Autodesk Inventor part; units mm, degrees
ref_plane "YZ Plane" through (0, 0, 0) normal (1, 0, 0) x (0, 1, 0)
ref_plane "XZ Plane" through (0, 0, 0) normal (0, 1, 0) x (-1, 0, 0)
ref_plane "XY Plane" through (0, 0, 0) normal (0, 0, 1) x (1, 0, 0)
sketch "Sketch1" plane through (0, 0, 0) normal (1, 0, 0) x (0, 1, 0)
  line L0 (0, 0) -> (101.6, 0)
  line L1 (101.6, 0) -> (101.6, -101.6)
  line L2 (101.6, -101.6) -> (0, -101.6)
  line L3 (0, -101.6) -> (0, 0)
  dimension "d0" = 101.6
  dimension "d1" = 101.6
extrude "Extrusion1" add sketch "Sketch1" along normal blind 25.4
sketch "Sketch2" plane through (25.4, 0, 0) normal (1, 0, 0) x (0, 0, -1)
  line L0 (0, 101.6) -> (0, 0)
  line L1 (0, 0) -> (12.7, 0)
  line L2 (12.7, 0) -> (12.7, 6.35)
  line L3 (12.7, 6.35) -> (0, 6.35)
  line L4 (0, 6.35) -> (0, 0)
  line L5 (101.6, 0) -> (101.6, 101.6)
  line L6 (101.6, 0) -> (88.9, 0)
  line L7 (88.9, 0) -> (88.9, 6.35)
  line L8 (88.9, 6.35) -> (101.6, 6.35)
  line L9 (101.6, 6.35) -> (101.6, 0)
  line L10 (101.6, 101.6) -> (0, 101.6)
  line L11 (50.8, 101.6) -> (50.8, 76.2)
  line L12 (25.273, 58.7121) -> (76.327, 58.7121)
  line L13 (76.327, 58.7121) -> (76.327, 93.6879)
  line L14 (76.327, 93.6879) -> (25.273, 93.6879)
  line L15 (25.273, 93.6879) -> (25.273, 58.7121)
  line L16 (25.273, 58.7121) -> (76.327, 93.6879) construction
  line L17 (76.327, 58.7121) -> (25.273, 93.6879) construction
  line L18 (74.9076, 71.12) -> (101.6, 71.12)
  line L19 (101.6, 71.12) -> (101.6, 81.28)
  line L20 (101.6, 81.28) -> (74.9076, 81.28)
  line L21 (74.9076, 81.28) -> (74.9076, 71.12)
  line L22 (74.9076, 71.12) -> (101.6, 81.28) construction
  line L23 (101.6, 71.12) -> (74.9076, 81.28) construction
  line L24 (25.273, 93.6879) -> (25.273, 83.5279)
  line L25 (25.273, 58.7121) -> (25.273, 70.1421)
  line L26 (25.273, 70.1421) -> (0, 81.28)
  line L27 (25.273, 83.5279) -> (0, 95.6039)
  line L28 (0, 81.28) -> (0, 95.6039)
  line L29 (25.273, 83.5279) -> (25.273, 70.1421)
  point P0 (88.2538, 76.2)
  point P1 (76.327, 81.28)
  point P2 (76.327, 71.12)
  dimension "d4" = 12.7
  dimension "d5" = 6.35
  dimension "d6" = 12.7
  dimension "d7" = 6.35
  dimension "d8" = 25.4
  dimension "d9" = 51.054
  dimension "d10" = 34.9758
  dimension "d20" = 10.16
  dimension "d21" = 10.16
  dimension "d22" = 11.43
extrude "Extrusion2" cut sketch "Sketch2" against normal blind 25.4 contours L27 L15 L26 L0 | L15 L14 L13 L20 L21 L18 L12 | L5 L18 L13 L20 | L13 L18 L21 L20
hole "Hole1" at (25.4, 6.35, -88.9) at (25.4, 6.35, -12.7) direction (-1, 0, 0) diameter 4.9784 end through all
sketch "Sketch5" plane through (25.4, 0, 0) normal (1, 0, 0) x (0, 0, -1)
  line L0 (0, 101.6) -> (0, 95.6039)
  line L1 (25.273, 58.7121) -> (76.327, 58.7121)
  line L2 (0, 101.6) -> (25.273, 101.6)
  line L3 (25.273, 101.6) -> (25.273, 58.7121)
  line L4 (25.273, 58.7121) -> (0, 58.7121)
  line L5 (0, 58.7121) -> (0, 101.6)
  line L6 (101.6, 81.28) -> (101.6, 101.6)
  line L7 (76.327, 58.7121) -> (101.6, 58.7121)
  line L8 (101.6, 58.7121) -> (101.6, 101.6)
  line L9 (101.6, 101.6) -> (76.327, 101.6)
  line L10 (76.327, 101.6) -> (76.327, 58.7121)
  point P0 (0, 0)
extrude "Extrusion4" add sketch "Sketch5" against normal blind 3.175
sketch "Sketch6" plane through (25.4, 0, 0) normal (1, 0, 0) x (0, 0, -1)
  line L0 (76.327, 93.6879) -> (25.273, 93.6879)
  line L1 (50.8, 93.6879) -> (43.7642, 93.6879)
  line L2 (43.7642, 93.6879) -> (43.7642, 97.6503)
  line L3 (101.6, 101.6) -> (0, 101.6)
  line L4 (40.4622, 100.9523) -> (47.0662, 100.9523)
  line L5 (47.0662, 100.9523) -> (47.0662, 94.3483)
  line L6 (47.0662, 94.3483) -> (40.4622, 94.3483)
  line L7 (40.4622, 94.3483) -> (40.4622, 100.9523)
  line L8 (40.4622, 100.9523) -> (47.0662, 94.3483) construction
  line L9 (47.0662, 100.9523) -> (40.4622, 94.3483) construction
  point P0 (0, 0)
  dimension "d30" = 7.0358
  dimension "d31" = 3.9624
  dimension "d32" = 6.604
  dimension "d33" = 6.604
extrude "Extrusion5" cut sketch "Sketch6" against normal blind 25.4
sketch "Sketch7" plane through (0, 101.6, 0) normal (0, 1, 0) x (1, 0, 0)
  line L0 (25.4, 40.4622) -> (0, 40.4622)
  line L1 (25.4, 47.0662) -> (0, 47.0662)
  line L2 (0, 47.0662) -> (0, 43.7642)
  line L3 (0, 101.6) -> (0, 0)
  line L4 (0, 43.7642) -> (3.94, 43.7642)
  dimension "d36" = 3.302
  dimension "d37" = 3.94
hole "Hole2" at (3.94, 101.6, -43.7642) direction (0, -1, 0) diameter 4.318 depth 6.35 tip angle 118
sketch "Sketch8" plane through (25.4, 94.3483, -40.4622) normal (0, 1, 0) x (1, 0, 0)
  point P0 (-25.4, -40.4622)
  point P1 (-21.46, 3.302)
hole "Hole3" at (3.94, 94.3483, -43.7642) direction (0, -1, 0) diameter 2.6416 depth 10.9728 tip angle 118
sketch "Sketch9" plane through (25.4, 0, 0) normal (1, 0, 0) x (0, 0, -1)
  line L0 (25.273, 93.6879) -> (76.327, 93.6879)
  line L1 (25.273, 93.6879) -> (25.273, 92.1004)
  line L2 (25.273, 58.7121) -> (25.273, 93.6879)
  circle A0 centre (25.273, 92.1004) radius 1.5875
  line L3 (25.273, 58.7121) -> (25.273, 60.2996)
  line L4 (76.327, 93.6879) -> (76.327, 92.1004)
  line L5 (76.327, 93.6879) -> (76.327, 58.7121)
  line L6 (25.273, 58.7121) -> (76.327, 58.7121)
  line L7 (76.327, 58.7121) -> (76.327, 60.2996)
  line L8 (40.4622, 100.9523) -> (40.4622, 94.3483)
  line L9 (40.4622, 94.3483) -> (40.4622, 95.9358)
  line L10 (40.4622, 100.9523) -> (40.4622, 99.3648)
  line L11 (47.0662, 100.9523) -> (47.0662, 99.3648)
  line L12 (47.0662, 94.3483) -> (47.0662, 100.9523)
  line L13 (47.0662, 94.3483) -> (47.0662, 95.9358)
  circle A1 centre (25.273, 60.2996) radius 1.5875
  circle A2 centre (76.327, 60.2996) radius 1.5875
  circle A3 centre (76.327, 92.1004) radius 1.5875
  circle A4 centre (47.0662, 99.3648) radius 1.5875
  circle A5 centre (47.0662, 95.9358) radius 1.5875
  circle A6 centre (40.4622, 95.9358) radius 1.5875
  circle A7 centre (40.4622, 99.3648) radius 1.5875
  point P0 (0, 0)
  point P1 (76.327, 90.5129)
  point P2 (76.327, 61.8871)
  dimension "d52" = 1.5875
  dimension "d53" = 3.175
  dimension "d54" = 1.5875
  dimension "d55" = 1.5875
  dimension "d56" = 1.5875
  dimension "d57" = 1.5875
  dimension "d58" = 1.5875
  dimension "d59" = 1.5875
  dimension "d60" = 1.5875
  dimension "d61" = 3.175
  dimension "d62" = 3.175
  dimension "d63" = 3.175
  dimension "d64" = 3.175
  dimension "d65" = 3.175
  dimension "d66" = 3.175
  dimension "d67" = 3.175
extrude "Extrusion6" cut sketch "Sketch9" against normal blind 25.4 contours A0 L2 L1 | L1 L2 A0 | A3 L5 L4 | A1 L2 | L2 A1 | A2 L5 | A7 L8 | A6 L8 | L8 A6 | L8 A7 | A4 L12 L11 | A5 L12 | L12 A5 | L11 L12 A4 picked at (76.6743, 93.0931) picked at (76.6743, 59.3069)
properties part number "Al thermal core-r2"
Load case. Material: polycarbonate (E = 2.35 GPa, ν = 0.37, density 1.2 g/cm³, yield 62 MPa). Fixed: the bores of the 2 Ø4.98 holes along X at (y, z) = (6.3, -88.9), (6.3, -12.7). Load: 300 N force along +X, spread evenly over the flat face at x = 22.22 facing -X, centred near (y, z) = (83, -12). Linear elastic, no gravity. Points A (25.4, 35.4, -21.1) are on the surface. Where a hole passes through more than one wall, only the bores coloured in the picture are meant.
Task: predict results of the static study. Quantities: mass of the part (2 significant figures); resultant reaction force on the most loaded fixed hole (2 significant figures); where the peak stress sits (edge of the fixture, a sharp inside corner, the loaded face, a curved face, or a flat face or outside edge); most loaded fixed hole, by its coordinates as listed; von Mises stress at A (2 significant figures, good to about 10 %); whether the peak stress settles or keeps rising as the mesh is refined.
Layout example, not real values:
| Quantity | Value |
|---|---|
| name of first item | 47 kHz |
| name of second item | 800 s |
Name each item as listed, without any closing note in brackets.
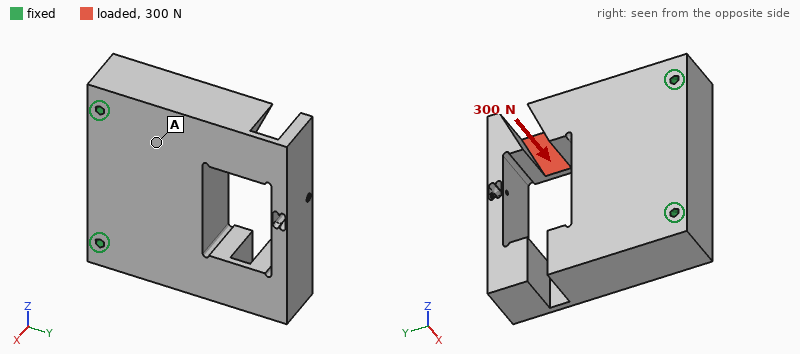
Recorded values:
| Quantity | Value |
|---|---|
| mass of the part | 240 g |
| resultant reaction force on the most loaded fixed hole | 280 N |
| where the peak stress sits | edge of the fixture |
| most loaded fixed hole, by its coordinates as listed | (6.3, -12.7) |
| von Mises stress at A | 2.6 MPa |
| whether the peak stress settles or keeps rising as the mesh is refined | keeps rising |
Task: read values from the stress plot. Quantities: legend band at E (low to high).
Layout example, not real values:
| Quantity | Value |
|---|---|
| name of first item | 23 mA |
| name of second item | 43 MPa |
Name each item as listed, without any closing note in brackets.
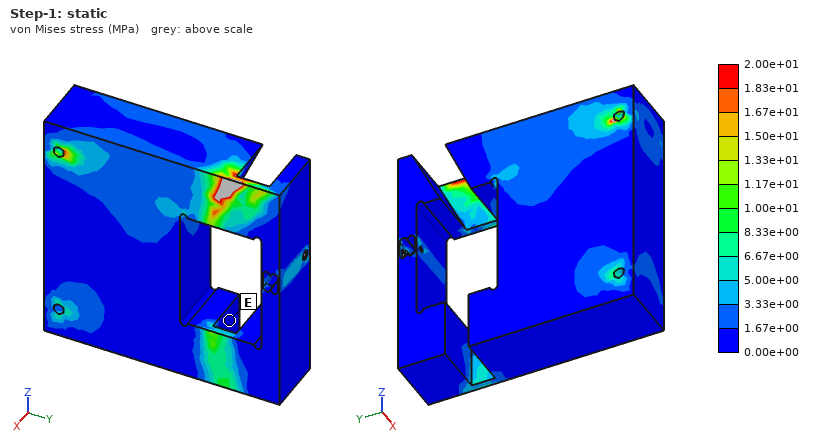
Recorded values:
| Quantity | Value |
|---|---|
| legend band at E | 0.00e+00 to 1.67e+00 MPa |
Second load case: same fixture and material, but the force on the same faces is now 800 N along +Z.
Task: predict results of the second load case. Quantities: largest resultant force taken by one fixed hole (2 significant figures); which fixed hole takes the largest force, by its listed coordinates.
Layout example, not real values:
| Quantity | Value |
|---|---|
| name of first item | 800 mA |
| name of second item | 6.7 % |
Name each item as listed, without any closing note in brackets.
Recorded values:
| Quantity | Value |
|---|---|
| largest resultant force taken by one fixed hole | 930 N |
| which fixed hole takes the largest force, by its listed coordinates | (6.3, -88.9) |
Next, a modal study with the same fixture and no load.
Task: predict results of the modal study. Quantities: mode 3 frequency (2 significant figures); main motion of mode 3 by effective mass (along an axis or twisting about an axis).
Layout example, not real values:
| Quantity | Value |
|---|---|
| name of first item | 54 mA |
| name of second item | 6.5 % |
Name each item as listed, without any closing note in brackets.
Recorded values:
| Quantity | Value |
|---|---|
| mode 3 frequency | 700 Hz |
| main motion of mode 3 by effective mass | along X |
